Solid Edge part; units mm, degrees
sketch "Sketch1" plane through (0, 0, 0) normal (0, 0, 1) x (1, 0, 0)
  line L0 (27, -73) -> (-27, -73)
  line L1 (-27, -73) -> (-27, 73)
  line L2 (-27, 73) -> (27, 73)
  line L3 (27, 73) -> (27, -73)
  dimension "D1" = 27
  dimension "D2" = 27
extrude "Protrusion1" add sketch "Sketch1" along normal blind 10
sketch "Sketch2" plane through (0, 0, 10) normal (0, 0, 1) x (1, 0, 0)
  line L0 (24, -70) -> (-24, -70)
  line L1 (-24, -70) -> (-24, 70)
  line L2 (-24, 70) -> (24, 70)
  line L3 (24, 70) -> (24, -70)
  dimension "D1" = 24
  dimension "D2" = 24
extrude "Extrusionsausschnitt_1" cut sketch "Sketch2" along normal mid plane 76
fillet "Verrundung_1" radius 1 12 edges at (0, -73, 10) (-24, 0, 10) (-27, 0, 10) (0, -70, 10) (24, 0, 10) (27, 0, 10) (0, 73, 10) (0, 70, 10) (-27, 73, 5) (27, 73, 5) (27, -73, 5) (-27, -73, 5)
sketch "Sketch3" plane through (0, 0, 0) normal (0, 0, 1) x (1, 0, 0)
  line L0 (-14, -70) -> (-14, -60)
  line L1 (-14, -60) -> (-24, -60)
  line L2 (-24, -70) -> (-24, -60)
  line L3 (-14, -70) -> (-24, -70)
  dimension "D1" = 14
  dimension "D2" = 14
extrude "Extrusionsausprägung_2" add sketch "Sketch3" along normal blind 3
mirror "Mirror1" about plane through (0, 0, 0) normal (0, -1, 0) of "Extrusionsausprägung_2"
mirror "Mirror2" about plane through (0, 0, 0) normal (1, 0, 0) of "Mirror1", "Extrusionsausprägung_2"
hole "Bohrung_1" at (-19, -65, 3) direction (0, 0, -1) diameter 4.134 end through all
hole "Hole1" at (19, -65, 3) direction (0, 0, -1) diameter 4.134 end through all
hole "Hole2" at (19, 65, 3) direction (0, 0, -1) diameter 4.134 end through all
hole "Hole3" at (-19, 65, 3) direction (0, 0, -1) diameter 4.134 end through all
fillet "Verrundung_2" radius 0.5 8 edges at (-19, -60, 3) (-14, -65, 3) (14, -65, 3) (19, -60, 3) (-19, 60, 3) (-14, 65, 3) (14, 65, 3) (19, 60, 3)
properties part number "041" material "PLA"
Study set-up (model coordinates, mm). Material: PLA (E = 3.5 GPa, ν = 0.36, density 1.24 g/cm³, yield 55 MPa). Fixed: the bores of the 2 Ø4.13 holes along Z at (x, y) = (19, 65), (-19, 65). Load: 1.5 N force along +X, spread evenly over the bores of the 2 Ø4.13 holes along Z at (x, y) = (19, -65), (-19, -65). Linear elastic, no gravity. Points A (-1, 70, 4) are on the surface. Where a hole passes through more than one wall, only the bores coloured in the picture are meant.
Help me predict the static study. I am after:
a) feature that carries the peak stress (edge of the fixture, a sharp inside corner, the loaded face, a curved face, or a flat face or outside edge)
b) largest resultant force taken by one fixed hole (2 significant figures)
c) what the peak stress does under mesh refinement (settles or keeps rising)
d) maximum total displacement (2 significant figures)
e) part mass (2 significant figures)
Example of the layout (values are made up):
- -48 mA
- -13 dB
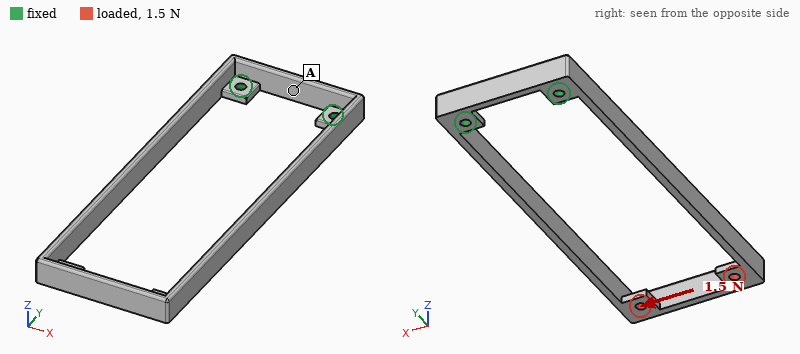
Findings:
- a sharp inside corner
- 2.2 N
- keeps rising
- 1.8 mm
- 15 g
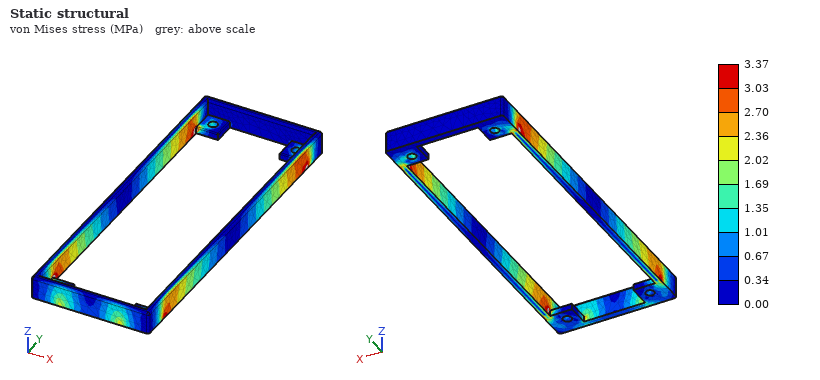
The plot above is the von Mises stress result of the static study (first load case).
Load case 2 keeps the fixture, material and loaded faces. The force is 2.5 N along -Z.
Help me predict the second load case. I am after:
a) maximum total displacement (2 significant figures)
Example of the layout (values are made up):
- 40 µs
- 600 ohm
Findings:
- 1.7 mm
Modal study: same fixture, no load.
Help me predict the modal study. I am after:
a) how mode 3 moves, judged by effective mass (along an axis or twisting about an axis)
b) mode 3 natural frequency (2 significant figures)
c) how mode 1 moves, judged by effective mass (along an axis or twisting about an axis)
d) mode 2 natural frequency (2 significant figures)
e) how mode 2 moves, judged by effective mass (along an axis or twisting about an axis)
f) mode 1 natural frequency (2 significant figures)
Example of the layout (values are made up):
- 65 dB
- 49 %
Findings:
- twisting about Y
- 160 Hz
- along X
- 84 Hz
- along Z
- 57 Hz
